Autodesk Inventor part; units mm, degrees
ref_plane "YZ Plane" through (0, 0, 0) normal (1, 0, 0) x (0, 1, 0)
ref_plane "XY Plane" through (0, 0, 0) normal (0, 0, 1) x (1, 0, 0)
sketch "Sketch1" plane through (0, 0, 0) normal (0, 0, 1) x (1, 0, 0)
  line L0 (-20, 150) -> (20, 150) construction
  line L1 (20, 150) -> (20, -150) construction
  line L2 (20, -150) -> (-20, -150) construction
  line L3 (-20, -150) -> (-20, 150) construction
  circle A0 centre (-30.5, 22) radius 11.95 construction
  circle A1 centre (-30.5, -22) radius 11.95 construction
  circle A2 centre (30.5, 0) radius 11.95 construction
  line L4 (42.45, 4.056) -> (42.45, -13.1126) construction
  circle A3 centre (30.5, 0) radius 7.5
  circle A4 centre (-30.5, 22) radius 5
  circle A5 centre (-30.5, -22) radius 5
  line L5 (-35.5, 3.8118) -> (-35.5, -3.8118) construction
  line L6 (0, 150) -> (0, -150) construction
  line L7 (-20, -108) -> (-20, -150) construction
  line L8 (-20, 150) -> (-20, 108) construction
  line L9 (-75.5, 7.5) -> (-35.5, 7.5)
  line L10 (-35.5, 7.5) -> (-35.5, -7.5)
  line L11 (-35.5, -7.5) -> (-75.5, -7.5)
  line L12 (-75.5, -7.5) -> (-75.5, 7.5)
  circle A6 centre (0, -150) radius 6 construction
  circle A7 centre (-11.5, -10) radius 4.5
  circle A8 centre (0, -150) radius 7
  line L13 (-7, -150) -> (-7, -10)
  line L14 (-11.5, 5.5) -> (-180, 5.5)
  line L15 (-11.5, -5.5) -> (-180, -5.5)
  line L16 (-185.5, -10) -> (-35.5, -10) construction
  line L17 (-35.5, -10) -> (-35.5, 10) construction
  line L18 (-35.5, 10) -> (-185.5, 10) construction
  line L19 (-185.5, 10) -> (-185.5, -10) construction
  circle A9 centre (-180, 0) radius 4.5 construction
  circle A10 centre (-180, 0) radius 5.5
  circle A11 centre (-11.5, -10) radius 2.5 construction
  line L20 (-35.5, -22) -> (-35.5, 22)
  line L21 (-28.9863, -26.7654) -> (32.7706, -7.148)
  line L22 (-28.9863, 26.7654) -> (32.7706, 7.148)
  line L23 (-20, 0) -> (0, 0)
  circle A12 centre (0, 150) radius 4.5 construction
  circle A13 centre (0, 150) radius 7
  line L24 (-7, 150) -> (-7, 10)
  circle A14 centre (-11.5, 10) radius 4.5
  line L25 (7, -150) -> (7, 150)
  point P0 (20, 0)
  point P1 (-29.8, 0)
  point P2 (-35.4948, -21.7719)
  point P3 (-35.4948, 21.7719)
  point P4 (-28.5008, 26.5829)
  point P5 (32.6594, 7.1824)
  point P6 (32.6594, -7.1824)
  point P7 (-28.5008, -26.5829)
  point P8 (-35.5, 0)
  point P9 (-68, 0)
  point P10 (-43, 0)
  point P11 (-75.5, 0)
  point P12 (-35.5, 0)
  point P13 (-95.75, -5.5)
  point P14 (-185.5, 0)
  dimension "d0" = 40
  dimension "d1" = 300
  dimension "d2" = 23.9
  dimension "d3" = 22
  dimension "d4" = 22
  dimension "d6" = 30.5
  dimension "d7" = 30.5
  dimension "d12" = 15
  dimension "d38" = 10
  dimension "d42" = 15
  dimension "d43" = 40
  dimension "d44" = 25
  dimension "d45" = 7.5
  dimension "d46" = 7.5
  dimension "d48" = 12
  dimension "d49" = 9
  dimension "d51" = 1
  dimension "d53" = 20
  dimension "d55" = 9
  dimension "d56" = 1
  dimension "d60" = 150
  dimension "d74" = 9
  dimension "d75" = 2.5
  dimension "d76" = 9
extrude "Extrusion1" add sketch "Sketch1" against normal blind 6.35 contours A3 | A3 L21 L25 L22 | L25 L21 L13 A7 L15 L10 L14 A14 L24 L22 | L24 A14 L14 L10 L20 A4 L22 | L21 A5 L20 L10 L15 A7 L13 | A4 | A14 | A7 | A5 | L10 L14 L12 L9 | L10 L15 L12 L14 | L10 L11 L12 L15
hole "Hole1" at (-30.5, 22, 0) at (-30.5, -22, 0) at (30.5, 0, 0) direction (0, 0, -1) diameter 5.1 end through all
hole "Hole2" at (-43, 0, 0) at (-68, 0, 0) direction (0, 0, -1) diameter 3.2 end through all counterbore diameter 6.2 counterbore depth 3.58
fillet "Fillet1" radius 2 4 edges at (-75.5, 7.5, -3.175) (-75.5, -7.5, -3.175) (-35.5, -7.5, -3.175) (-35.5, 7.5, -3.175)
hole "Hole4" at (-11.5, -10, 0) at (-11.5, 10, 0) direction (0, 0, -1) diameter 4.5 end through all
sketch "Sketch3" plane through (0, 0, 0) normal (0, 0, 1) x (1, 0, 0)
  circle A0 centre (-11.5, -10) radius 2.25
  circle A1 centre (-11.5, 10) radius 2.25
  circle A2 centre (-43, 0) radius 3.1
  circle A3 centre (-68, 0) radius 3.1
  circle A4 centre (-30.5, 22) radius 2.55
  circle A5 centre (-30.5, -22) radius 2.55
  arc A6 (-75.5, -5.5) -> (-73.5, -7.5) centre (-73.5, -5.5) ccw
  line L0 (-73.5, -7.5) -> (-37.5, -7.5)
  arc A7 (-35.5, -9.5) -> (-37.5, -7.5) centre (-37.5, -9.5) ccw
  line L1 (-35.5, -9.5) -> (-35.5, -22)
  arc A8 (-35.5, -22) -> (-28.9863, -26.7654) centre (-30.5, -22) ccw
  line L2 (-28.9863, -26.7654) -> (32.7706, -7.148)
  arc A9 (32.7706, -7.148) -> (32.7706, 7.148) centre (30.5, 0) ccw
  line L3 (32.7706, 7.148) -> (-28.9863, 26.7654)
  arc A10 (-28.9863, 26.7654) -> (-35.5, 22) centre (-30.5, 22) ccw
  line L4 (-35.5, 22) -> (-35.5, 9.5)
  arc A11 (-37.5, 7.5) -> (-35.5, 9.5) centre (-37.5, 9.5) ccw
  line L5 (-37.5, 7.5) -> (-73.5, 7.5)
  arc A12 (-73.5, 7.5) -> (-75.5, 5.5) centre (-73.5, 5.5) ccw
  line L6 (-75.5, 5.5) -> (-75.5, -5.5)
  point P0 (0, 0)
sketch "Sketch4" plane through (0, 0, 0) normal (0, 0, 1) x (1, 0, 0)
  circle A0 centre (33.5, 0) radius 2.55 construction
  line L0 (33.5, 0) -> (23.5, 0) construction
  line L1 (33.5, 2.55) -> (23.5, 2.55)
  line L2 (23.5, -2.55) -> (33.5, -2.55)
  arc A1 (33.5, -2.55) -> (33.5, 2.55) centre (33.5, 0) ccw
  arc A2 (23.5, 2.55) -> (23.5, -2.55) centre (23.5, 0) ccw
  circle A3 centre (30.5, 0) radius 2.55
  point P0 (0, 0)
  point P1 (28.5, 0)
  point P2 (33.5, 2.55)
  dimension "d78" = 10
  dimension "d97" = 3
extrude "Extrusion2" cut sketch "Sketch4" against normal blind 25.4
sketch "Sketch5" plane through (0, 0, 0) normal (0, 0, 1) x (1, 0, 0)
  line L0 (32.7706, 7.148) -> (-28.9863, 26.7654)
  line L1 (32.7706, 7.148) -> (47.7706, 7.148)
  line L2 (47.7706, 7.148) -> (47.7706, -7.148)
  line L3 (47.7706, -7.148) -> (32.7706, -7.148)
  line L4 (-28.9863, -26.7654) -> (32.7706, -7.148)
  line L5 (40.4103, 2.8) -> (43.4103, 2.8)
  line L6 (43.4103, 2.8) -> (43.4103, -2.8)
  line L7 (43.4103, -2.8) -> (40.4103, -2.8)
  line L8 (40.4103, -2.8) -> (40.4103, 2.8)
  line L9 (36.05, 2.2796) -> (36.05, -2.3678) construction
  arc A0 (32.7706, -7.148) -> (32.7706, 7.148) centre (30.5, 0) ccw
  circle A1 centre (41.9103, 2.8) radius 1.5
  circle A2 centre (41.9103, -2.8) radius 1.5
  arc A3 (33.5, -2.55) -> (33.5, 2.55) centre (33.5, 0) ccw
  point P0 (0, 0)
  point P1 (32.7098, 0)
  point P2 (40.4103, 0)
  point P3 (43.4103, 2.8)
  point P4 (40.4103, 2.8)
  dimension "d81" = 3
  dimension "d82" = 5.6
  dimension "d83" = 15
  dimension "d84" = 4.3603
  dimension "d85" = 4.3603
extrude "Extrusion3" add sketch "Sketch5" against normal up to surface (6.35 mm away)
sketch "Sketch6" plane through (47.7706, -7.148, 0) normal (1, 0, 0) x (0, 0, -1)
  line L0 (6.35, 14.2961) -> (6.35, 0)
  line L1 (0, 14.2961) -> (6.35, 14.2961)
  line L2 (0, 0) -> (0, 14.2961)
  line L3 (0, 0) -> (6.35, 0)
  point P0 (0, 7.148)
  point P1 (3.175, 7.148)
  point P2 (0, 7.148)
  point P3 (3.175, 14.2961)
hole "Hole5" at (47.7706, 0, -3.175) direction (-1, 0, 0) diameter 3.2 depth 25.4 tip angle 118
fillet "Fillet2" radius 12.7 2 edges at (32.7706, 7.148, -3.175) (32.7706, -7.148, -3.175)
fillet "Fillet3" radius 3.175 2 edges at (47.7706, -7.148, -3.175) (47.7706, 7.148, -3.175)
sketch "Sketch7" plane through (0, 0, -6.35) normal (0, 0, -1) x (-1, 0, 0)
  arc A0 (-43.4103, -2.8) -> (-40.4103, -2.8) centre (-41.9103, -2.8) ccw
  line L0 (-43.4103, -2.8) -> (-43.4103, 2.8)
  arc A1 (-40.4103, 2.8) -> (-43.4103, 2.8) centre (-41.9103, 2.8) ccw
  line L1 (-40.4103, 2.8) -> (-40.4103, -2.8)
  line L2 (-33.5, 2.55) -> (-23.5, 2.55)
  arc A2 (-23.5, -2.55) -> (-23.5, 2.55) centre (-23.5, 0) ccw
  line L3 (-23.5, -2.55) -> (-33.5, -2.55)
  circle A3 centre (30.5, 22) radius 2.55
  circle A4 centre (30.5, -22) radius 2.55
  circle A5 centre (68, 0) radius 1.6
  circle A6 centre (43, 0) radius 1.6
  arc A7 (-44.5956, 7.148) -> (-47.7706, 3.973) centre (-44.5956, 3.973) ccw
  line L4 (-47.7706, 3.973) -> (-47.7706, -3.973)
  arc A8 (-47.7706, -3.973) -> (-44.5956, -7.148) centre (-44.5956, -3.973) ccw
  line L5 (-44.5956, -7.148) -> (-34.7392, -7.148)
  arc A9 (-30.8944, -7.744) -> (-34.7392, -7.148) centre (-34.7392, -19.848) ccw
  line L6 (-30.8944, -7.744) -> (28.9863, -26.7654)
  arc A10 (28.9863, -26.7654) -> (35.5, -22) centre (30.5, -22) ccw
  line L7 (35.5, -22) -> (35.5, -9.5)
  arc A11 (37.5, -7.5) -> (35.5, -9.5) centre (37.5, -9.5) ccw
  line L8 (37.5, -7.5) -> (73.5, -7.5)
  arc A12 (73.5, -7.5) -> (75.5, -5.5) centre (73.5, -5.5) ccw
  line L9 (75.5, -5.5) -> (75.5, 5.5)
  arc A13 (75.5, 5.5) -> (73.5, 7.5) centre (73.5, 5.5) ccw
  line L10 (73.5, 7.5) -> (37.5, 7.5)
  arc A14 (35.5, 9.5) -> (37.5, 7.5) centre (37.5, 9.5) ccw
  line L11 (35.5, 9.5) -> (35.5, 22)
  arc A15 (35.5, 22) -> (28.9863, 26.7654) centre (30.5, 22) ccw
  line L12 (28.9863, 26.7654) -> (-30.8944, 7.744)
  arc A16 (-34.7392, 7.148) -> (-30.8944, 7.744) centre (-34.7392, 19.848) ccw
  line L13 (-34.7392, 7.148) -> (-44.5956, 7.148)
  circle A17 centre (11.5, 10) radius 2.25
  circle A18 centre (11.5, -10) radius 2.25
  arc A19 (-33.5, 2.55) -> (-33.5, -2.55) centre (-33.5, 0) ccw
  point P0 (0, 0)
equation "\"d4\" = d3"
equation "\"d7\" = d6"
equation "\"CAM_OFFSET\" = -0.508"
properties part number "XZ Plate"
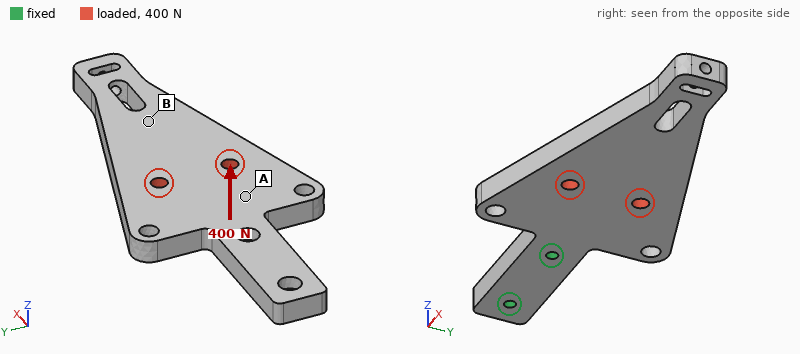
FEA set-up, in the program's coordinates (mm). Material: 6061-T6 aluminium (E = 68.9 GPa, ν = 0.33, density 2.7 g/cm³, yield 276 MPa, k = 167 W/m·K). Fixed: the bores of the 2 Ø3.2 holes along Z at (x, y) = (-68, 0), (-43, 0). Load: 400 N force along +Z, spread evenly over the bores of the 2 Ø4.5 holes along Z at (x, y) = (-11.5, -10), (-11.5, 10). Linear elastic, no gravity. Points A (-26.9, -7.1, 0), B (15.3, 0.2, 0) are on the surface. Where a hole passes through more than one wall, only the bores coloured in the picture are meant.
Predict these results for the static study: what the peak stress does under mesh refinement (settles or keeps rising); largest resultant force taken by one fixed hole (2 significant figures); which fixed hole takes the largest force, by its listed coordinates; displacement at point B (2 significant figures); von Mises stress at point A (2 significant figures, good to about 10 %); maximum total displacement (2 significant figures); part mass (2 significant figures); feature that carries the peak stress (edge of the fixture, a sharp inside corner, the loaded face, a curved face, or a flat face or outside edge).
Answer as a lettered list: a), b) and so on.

a) keeps rising
b) 1.1 kN
c) (-43, 0)
d) 0.52 mm
e) 27 MPa
f) 0.83 mm
g) 52 g
h) edge of the fixture
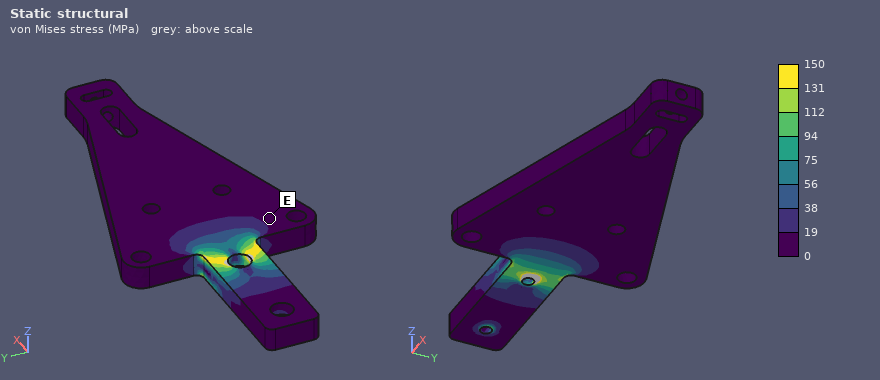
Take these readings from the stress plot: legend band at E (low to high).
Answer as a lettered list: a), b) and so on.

a) 0 to 19 MPa
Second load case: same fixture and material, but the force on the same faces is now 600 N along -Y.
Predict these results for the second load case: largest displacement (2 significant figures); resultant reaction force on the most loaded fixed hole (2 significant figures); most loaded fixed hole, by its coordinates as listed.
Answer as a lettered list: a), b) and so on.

a) 0.28 mm
b) 1.2 kN
c) (-43, 0)
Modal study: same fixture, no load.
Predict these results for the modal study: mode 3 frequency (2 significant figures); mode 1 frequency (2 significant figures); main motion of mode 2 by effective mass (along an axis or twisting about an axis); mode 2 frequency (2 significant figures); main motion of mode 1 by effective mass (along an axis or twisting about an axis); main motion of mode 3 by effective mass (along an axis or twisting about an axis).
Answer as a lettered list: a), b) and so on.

a) 2100 Hz
b) 630 Hz
c) along Y
d) 1300 Hz
e) along Z
f) twisting about X
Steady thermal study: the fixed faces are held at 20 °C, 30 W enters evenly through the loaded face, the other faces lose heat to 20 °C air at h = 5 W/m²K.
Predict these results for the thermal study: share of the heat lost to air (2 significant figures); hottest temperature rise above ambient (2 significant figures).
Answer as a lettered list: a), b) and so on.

a) 4.6 %
b) 44 K
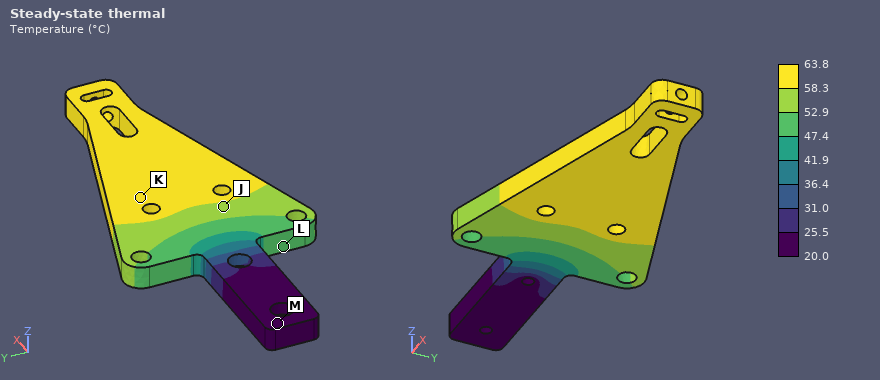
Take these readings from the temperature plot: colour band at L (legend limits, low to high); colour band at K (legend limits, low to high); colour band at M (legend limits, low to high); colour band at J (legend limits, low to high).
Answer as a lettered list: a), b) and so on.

a) 47.4 to 52.9 °C
b) 58.3 to 63.8 °C
c) 20.0 to 25.5 °C
d) 52.9 to 58.3 °C
